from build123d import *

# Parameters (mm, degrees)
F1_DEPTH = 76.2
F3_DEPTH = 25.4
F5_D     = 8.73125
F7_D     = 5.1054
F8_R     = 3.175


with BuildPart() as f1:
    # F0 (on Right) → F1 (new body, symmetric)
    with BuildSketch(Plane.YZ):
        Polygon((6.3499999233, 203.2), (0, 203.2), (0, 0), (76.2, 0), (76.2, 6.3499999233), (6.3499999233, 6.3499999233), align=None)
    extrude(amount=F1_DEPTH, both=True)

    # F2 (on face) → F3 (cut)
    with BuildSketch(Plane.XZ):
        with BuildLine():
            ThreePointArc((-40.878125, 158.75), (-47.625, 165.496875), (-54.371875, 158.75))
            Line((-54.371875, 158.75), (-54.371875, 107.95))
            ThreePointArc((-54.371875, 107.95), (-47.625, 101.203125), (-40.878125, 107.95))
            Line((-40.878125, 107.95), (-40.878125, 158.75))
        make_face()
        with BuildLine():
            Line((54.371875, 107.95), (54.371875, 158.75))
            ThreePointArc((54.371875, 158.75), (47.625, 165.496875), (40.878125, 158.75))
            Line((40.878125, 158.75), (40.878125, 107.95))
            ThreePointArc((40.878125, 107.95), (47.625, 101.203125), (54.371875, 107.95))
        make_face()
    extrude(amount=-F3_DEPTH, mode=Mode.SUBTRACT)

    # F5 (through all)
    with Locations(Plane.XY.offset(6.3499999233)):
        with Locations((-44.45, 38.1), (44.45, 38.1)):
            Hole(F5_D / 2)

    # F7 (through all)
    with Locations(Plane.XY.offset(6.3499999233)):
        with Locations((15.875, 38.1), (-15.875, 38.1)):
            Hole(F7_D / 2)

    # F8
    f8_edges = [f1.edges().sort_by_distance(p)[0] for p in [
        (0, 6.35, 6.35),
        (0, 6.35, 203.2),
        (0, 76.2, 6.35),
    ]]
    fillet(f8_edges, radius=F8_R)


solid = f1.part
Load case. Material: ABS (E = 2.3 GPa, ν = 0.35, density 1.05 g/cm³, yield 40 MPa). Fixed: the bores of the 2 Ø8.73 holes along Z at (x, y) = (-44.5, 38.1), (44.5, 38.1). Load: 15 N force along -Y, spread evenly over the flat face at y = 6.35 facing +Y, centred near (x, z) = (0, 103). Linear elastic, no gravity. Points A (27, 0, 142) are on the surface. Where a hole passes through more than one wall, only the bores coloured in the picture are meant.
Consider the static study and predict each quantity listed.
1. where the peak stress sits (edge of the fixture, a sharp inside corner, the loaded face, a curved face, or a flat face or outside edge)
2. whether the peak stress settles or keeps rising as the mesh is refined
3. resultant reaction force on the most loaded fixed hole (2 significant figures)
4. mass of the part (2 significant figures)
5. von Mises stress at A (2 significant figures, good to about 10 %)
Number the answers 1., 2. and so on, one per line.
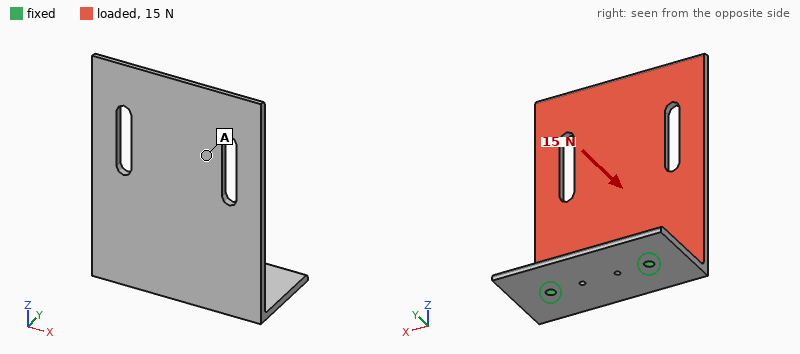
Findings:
1. edge of the fixture
2. keeps rising
3. 7.8 N
4. 260 g
5. 0.17 MPa
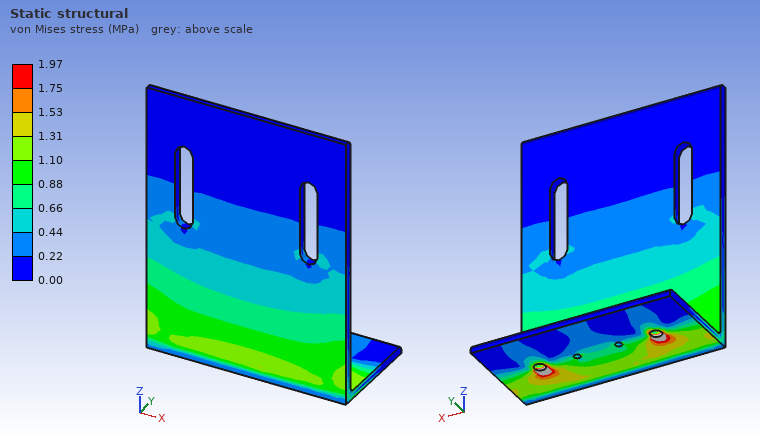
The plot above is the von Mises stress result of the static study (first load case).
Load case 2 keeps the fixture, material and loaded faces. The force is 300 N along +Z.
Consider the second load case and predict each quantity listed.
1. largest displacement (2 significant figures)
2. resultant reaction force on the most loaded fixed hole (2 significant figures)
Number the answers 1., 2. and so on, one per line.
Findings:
1. 3.1 mm
2. 150 N
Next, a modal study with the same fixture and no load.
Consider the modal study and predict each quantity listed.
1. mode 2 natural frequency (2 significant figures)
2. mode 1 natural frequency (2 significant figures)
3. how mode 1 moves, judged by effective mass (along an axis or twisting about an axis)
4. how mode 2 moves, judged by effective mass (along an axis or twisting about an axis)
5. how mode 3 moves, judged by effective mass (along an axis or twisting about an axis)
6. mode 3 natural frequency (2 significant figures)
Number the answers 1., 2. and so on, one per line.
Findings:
1. 99 Hz
2. 31 Hz
3. along Y
4. along X
5. along X
6. 140 Hz
